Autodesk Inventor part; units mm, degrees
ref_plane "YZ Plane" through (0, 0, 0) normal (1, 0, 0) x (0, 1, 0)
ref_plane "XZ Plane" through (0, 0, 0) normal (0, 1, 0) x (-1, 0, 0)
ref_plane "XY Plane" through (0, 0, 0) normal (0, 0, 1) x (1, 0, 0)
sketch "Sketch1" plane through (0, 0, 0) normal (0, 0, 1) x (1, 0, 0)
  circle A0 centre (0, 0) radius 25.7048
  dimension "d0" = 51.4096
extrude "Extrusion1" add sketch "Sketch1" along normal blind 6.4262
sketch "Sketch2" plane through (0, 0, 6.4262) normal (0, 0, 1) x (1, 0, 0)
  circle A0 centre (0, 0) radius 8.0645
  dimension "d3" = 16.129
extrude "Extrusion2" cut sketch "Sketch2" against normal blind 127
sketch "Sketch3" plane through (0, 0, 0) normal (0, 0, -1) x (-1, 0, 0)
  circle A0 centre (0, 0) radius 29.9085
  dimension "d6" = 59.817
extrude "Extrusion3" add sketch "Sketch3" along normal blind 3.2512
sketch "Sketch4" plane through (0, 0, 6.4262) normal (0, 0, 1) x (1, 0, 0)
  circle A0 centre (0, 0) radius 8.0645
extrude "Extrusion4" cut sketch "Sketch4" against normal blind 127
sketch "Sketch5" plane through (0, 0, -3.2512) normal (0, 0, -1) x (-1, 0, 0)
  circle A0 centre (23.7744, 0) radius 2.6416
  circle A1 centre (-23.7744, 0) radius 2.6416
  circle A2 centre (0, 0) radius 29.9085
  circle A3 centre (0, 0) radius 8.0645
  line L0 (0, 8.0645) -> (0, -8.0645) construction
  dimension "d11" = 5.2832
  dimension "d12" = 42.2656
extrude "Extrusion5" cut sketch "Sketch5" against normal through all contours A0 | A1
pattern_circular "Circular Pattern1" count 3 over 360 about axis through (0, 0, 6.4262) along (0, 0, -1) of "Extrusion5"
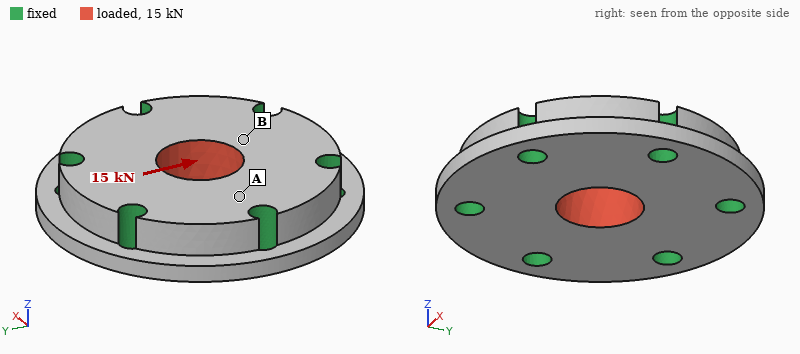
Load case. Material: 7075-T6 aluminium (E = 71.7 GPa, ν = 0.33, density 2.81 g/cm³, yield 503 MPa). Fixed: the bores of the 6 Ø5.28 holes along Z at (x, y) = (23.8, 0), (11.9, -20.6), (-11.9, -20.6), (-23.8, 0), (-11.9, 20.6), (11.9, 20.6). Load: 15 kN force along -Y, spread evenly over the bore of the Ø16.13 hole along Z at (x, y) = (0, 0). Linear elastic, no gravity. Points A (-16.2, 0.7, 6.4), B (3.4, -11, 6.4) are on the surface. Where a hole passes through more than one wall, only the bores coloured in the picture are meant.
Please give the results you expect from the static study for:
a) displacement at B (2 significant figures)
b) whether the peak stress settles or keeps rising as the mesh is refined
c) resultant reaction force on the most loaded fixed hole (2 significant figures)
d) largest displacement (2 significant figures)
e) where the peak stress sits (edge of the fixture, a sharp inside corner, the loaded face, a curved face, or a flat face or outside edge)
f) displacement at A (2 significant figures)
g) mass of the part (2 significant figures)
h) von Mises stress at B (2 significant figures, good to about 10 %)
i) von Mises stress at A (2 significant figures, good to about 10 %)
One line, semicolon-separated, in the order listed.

5.5 µm; keeps rising; 3.4 kN; 7.2 µm; edge of the fixture; 2.0 µm; 54 g; 28 MPa; 7.6 MPa
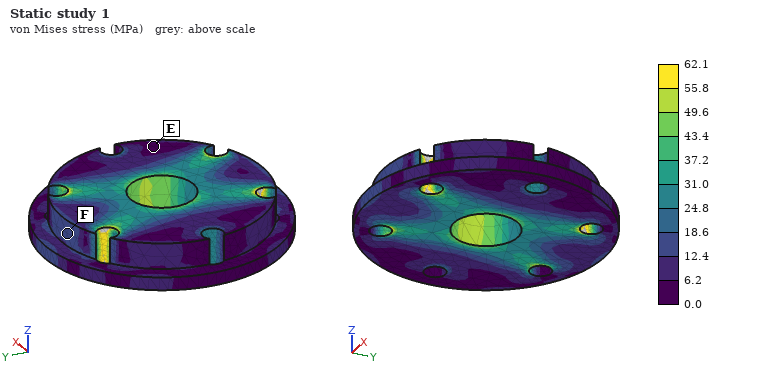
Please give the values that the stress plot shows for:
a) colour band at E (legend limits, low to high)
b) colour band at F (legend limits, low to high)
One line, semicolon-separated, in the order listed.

0.0 to 6.2 MPa; 12.4 to 18.6 MPa
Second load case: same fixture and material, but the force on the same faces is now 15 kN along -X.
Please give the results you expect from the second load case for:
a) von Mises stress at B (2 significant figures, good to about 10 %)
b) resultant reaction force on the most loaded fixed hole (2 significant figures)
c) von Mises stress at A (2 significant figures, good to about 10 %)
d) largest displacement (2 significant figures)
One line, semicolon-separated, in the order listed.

25 MPa; 3.9 kN; 39 MPa; 7.1 µm
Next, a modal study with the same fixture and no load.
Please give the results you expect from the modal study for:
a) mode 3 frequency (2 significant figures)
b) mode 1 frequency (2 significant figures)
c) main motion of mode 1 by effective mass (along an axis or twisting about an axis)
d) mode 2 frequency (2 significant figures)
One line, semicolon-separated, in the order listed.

45 kHz; 32 kHz; along Z; 45 kHz
